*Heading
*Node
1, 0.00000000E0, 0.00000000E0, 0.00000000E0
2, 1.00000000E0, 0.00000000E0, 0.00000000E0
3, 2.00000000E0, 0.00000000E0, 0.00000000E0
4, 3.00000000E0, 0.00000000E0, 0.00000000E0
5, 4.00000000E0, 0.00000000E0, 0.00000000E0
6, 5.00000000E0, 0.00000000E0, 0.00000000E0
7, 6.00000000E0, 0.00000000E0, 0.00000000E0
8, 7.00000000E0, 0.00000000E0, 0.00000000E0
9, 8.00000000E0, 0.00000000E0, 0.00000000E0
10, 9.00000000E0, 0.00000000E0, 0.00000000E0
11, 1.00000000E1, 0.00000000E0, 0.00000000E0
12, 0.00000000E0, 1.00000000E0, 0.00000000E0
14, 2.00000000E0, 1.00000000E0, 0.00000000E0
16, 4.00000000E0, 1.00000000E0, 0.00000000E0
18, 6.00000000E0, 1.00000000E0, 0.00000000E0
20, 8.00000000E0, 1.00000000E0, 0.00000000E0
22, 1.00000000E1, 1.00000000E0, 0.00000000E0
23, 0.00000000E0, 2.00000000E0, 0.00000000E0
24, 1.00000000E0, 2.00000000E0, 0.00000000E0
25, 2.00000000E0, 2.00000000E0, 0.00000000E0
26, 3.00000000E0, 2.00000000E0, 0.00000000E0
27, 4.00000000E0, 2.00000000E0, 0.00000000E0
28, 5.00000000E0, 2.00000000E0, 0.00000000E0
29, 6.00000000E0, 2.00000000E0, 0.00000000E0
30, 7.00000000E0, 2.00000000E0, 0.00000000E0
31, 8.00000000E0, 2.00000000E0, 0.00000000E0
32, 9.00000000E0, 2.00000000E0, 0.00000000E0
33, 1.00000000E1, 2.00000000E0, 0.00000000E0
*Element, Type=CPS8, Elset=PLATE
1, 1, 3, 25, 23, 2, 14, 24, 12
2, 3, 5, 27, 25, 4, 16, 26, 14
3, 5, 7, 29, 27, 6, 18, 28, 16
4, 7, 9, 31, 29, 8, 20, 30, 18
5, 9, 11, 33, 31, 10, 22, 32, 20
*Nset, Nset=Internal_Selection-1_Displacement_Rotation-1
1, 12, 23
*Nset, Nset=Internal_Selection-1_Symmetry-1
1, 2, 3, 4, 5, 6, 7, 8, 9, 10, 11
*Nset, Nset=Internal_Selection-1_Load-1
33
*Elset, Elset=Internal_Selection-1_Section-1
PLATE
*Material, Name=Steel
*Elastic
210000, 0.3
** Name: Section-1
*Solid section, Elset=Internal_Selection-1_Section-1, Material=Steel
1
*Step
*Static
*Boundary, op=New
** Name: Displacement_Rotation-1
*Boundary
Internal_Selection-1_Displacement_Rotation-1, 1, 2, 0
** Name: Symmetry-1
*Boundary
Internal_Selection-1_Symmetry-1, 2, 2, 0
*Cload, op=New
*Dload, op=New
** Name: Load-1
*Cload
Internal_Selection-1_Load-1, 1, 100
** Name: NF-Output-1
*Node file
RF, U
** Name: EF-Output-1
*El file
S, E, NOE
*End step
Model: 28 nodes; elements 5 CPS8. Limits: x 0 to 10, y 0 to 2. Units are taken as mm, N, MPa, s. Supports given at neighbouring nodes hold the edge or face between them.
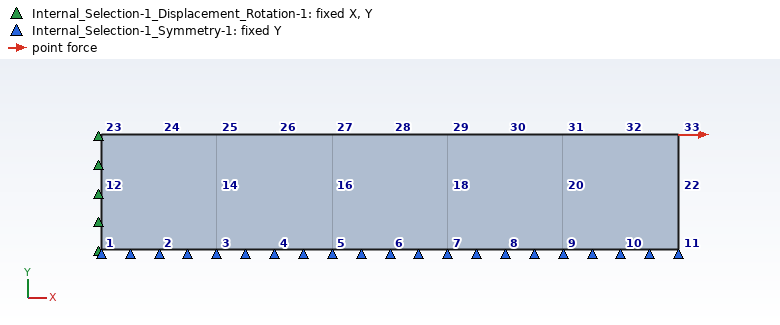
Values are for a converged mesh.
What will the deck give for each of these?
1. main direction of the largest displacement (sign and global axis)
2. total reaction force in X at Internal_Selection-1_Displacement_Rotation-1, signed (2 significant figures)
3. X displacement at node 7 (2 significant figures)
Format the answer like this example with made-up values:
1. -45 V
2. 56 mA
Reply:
1. +X
2. -100 N
3. 0.0014 mm
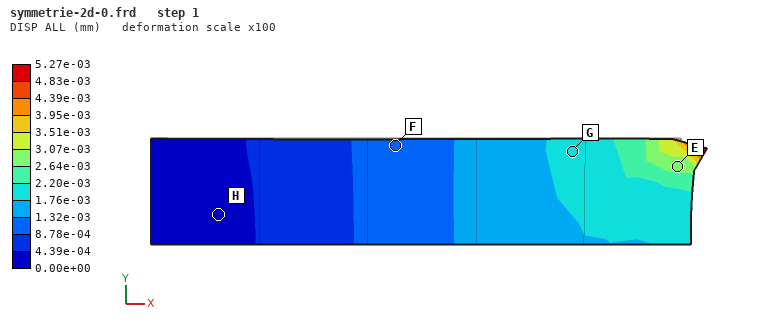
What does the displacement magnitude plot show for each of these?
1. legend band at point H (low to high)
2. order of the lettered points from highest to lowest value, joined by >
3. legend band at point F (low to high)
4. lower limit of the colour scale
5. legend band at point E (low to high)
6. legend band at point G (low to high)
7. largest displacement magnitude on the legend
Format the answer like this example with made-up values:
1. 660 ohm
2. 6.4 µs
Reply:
1. 0.00e+00 to 4.39e-04 mm
2. E > G > F > H
3. 8.78e-04 to 1.32e-03 mm
4. 0.00e+00 mm
5. 2.64e-03 to 3.07e-03 mm
6. 1.76e-03 to 2.20e-03 mm
7. 5.27e-03 mm
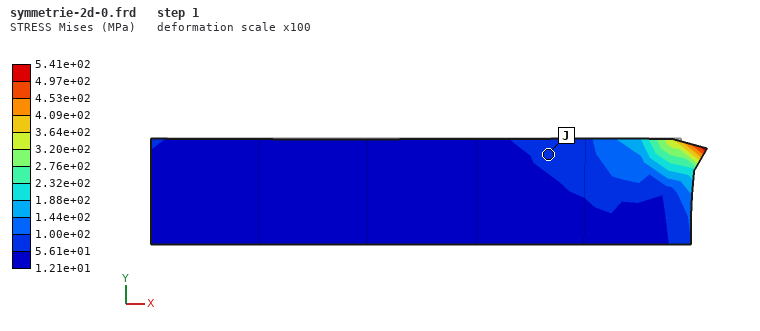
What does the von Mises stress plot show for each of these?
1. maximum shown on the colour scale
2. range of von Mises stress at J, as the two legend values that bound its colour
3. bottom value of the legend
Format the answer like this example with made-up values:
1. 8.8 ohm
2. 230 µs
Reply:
1. 5.41e+02 MPa
2. 5.61e+01 to 1.00e+02 MPa
3. 1.21e+01 MPa
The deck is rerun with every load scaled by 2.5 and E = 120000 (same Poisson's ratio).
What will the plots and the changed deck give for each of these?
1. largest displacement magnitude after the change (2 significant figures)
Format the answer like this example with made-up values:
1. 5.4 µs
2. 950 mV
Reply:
1. 0.023 mm
